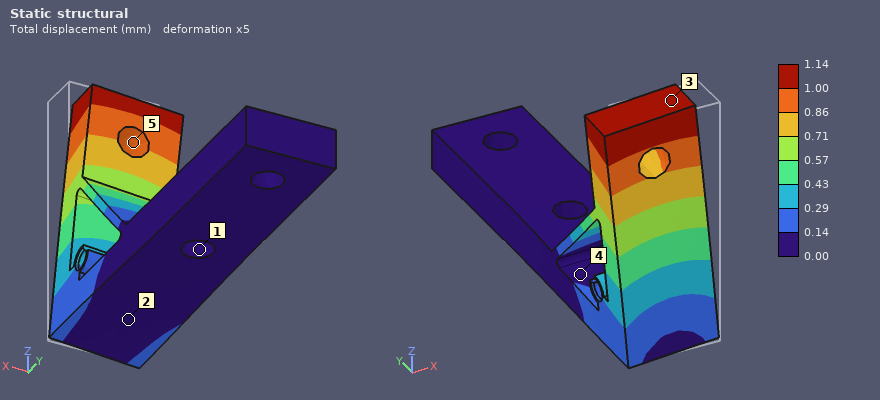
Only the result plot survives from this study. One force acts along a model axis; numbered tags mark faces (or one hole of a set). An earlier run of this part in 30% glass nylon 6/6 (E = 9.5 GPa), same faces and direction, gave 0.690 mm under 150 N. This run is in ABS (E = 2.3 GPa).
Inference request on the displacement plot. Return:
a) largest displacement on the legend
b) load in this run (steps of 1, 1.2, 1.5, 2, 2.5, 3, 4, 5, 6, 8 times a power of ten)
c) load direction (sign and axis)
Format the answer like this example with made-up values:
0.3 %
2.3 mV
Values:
1.14 mm
60 N
-X
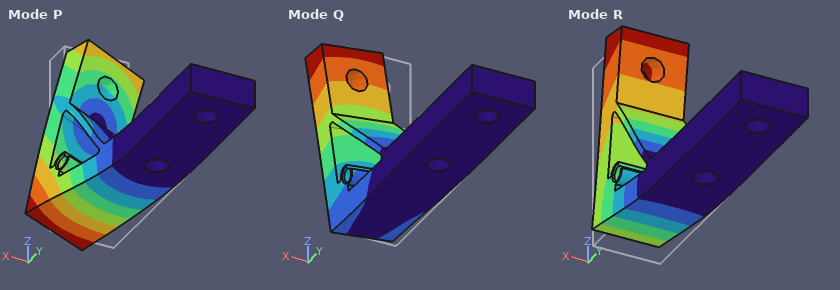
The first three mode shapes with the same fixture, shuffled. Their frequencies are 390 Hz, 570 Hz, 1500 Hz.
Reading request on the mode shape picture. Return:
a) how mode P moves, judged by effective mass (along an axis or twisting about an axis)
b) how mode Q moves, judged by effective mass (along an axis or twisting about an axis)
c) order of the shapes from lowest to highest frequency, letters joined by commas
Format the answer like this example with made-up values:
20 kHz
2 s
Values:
along X
along X
R, Q, P
